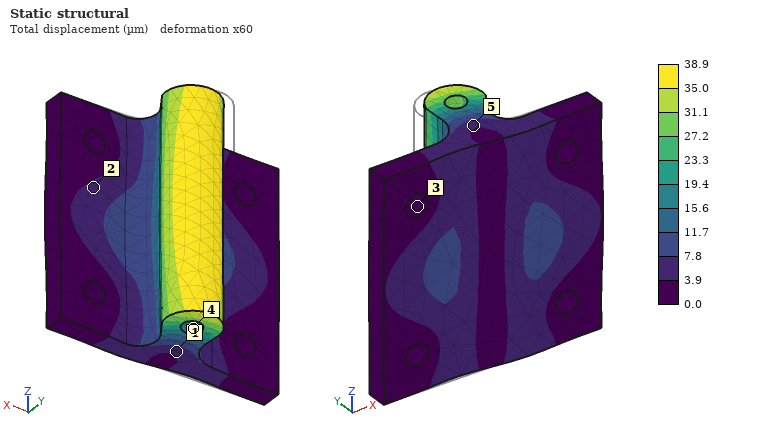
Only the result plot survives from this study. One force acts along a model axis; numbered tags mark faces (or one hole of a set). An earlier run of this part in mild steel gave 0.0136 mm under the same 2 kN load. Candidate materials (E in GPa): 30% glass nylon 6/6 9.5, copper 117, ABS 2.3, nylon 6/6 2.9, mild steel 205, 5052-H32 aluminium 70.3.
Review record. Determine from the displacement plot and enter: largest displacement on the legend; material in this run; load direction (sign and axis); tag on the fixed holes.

38.9 µm
5052-H32 aluminium
+X
3
